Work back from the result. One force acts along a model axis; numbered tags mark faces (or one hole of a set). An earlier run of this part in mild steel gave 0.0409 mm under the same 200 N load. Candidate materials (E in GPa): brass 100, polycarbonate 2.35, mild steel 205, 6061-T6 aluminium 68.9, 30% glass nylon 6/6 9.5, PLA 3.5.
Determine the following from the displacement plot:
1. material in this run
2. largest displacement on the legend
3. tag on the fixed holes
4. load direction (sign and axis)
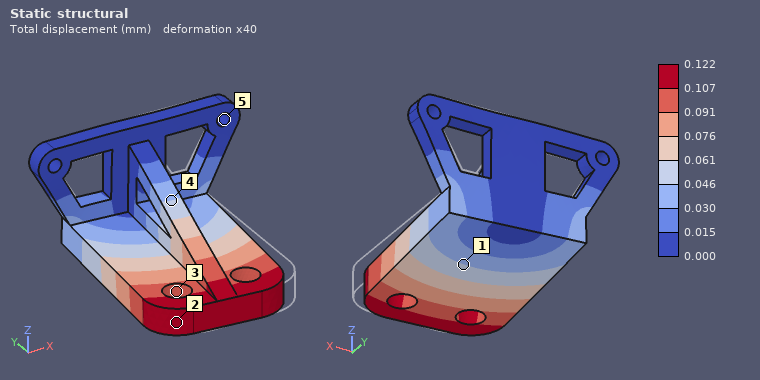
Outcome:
6061-T6 aluminium
0.122 mm
5
-X
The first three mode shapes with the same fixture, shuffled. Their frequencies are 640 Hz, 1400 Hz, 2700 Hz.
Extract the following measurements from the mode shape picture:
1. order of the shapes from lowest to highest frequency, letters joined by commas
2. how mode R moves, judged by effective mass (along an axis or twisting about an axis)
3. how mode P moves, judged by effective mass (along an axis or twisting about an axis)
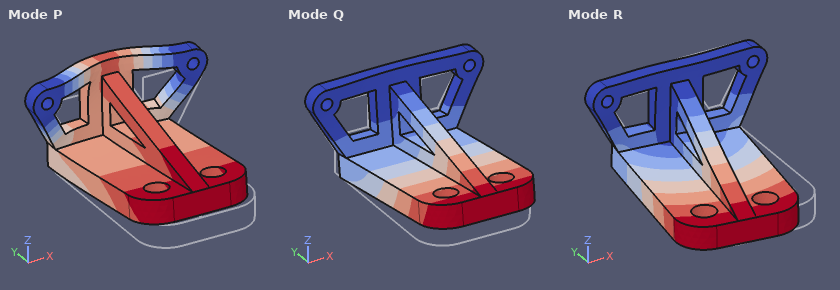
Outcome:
Q, R, P
along X
along Y
